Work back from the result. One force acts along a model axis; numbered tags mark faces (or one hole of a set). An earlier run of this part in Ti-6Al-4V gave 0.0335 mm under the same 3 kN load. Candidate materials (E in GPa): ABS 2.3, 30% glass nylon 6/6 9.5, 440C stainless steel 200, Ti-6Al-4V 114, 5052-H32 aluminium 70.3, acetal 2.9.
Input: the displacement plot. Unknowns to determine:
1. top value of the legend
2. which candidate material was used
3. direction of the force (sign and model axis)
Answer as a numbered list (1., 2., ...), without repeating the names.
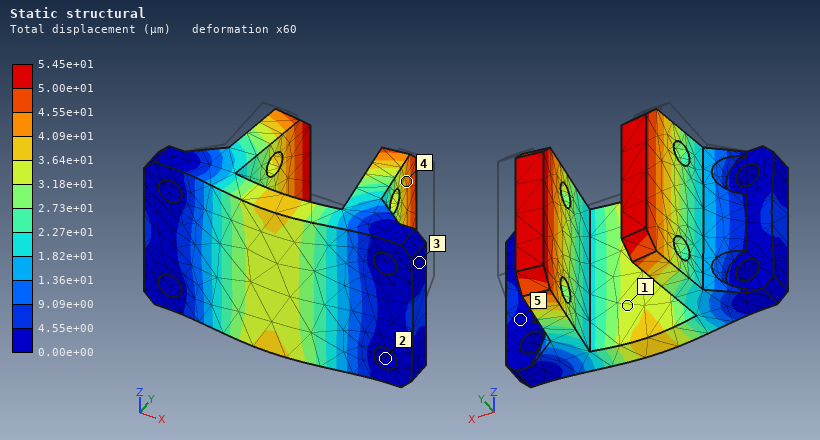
1. 5.45e+01 µm
2. 5052-H32 aluminium
3. -Y
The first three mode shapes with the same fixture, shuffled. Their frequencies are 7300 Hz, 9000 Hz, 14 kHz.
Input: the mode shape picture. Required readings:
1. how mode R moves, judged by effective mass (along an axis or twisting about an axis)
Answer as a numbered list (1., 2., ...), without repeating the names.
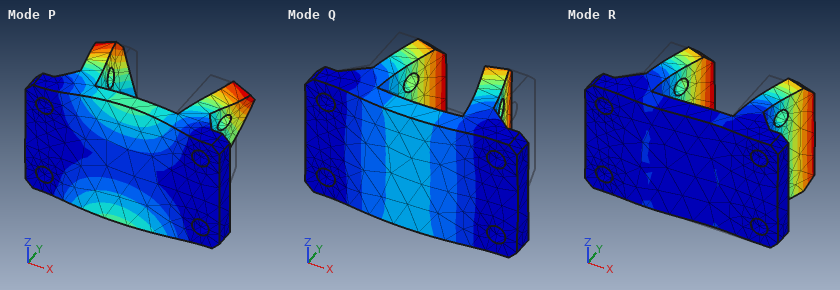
1. along X
